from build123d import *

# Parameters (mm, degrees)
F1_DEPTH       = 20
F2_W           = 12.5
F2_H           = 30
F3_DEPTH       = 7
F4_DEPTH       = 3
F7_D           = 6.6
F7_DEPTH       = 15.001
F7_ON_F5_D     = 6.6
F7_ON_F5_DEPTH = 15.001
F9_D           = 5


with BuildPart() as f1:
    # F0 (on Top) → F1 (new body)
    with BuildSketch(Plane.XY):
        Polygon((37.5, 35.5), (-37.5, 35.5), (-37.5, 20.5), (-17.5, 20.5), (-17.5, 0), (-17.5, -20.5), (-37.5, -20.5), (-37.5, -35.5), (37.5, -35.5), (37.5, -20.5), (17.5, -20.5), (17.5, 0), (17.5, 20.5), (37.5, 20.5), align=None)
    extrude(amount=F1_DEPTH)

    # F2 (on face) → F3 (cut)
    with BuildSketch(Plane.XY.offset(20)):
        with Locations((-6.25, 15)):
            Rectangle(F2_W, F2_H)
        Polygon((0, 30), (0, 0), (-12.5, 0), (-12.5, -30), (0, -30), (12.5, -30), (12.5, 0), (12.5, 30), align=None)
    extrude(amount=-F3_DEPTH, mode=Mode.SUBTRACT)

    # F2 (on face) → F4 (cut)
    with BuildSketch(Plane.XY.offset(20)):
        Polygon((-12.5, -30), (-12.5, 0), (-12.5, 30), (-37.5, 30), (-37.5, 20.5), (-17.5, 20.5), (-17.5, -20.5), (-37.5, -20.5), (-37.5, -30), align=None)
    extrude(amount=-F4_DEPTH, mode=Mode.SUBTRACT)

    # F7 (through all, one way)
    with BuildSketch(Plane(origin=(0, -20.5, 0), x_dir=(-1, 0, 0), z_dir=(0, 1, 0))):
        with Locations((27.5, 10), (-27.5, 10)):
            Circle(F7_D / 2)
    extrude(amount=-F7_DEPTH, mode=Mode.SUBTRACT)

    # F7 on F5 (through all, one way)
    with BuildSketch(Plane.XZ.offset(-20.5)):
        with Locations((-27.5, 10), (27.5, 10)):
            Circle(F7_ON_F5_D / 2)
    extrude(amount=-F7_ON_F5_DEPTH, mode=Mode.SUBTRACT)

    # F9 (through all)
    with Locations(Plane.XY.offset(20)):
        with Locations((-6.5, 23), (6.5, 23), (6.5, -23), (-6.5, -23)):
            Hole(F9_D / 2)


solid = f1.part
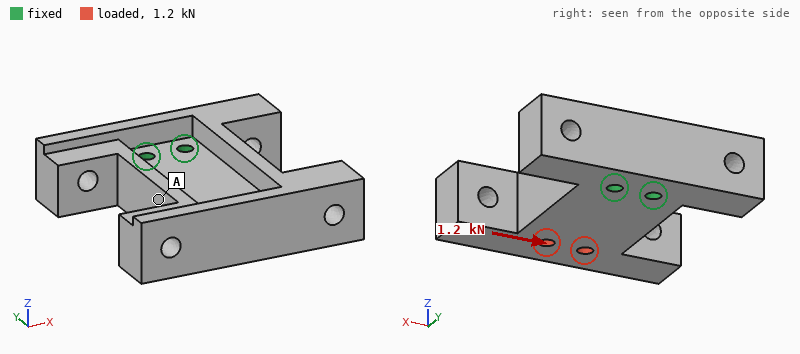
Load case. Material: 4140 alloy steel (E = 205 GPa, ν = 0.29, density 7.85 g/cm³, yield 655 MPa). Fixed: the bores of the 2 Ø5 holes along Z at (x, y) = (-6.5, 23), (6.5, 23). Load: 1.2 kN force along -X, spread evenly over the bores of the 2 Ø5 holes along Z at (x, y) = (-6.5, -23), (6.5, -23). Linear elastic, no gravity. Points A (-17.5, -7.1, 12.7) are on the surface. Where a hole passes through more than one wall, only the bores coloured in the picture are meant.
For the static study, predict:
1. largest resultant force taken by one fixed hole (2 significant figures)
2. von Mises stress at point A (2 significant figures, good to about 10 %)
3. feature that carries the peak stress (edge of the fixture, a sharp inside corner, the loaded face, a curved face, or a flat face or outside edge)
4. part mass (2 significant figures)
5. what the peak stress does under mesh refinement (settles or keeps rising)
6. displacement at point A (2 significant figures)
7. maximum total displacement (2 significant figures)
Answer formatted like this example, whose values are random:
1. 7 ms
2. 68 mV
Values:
1. 3.3 kN
2. 6.1 MPa
3. edge of the fixture
4. 460 g
5. keeps rising
6. 5.4 µm
7. 12 µm
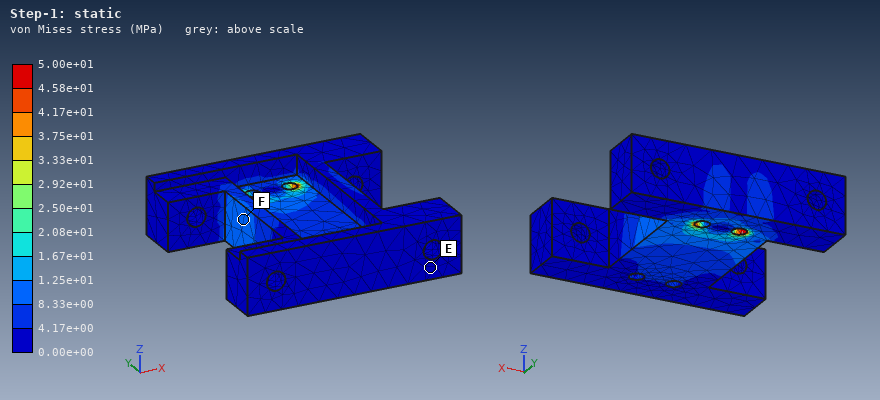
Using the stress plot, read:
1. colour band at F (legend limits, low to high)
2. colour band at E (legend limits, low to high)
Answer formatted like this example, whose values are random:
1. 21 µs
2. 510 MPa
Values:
1. 8.33e+00 to 1.25e+01 MPa
2. 0.00e+00 to 4.17e+00 MPa
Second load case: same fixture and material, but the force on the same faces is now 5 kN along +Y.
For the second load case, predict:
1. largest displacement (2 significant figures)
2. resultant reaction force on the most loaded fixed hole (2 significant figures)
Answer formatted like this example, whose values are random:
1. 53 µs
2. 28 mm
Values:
1. 4.1 µm
2. 2.5 kN
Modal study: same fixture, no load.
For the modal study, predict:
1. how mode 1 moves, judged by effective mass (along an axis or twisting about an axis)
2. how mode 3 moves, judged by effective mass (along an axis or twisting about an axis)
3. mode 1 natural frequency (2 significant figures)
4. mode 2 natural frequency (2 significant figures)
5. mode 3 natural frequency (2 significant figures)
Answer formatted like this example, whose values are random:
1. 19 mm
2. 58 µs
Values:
1. along Z
2. along X
3. 2300 Hz
4. 3200 Hz
5. 3800 Hz
